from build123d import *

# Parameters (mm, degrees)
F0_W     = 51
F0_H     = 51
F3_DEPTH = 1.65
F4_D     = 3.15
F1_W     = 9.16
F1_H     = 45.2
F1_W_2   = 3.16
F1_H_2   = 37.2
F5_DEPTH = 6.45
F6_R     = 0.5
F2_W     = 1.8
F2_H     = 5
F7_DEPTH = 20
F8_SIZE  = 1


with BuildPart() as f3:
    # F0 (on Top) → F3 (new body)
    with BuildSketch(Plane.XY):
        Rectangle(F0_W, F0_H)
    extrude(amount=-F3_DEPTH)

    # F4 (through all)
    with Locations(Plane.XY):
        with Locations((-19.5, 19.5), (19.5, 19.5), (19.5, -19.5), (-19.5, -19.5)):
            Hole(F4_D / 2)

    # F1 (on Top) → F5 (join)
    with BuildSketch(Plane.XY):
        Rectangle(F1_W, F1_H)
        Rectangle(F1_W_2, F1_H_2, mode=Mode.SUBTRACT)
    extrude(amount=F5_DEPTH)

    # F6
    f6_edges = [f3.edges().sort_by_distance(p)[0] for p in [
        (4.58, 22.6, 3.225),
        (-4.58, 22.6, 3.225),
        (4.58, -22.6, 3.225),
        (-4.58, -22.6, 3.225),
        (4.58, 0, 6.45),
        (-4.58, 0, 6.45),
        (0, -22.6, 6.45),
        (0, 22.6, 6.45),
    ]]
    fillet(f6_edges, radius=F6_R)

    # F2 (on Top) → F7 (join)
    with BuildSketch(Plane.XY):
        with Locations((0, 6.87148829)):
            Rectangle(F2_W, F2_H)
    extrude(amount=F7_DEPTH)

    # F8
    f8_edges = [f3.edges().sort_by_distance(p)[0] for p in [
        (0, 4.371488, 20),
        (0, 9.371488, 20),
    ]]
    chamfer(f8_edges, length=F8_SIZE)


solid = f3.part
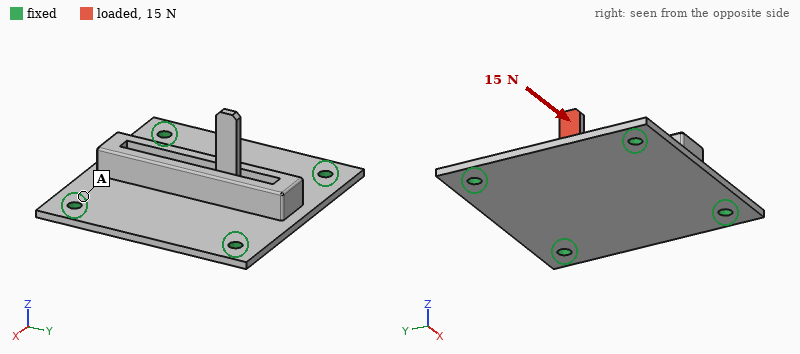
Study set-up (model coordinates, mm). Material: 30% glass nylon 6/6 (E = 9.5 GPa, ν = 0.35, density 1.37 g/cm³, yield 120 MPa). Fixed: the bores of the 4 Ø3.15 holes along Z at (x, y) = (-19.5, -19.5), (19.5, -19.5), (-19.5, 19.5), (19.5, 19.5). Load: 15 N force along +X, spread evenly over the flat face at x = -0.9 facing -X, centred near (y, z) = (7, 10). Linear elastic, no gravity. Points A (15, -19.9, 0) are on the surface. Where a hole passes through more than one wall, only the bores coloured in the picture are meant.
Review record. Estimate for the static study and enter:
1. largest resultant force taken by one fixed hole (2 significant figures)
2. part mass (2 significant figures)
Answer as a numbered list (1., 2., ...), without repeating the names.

1. 6.1 N
2. 8.7 g
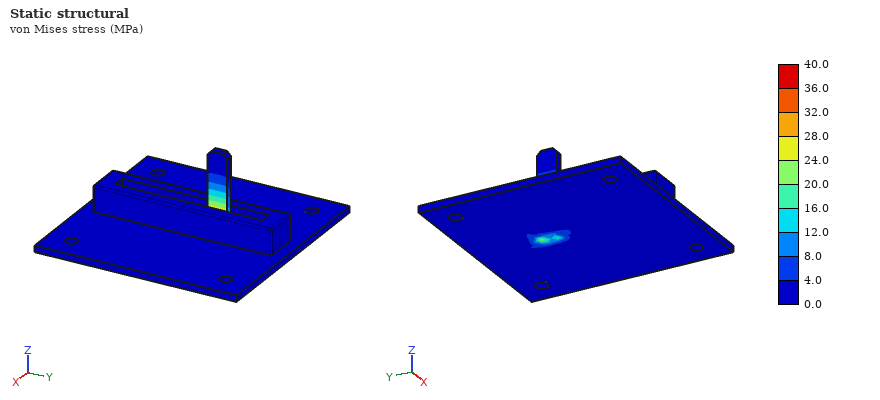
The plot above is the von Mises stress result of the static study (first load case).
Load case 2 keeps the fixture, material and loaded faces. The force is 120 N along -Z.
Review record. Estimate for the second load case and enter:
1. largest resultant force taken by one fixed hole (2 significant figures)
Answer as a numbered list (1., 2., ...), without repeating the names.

1. 46 N
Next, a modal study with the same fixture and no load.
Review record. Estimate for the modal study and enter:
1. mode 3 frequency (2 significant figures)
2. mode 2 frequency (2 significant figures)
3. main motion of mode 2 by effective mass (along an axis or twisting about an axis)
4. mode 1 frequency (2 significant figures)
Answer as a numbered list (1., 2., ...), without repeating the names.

1. 2600 Hz
2. 1900 Hz
3. along Z
4. 1800 Hz
